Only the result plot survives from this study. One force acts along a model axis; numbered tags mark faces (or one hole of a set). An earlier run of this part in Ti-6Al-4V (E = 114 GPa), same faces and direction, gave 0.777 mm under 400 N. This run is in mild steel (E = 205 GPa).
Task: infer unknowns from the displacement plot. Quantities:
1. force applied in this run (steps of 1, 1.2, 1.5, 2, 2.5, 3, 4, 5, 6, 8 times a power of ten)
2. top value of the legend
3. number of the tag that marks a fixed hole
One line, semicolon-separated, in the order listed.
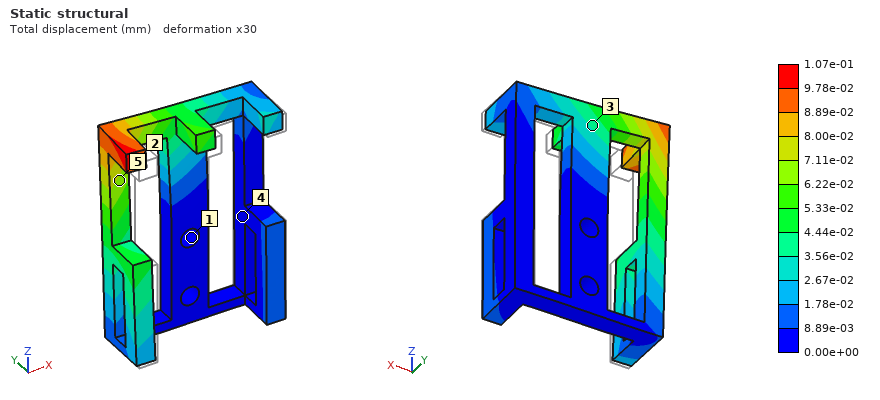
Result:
100 N; 1.07e-01 mm; 1
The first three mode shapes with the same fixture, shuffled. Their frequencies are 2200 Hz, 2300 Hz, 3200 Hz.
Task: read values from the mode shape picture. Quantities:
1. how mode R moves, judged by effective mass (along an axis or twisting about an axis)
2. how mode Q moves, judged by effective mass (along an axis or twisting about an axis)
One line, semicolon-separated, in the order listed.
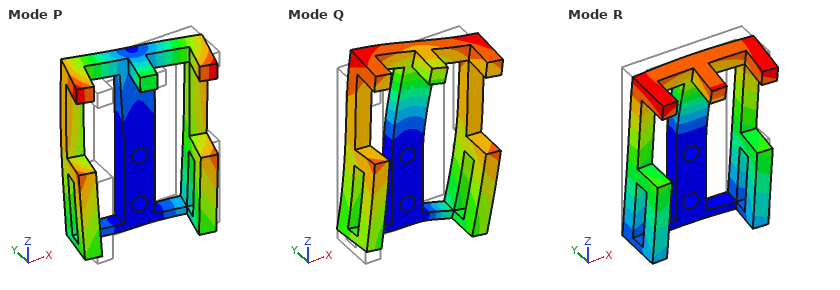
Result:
along Y; along X
